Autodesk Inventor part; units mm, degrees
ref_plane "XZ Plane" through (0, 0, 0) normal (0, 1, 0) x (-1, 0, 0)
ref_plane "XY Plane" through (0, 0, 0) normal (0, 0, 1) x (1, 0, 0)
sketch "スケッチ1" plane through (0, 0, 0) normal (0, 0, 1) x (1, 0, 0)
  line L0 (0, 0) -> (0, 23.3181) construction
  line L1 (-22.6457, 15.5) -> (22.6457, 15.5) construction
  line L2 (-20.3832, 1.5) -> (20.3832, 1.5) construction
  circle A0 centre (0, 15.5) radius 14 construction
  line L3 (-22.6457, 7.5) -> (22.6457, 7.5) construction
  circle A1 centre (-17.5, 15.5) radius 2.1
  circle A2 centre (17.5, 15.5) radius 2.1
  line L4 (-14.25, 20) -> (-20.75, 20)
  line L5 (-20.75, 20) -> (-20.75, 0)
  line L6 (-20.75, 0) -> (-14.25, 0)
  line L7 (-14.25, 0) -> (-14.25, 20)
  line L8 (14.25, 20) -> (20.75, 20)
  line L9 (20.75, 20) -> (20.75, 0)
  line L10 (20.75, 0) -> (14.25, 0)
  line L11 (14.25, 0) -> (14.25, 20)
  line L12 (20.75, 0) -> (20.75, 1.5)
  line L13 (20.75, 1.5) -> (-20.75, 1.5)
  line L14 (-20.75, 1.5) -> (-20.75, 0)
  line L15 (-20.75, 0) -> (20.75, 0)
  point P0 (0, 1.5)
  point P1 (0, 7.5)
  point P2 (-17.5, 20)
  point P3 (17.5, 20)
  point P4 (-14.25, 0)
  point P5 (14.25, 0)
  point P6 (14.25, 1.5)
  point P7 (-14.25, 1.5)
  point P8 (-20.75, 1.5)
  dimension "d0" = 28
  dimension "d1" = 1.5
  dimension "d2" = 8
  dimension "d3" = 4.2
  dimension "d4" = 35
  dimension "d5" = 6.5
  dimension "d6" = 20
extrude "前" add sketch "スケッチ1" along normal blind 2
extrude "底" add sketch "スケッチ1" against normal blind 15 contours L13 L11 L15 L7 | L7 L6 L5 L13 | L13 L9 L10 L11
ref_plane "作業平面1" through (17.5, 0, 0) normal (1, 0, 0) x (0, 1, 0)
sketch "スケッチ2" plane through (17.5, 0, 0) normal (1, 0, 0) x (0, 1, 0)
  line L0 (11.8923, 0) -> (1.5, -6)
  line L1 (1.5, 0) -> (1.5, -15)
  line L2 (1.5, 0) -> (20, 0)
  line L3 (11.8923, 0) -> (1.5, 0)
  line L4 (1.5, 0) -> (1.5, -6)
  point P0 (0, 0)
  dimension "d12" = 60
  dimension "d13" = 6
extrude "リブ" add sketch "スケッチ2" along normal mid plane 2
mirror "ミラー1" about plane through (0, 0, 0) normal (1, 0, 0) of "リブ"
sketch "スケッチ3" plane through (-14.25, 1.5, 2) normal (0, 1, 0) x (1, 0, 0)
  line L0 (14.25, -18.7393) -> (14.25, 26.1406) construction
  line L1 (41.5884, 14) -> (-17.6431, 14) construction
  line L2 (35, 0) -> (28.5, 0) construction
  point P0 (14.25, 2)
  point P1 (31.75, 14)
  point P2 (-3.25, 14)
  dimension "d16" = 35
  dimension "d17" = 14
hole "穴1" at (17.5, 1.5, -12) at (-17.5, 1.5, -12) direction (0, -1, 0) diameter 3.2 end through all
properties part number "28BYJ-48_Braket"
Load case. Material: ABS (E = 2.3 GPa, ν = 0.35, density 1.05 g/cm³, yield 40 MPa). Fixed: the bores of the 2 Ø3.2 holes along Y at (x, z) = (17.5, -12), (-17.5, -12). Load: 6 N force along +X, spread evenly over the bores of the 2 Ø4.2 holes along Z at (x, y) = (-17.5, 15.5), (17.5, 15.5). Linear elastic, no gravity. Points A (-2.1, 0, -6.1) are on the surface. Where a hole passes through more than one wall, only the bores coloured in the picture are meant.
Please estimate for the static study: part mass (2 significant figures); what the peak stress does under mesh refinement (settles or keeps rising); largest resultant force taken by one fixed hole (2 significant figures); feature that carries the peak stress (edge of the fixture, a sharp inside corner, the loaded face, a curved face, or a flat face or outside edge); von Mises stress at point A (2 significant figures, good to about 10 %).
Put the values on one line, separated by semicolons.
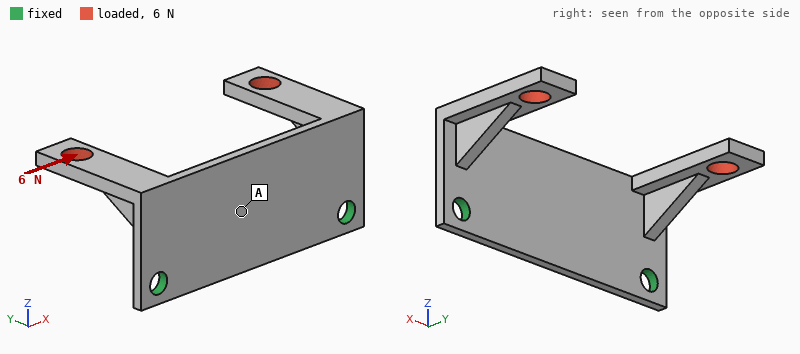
1.7 g; keeps rising; 3.8 N; edge of the fixture; 1.0 MPa
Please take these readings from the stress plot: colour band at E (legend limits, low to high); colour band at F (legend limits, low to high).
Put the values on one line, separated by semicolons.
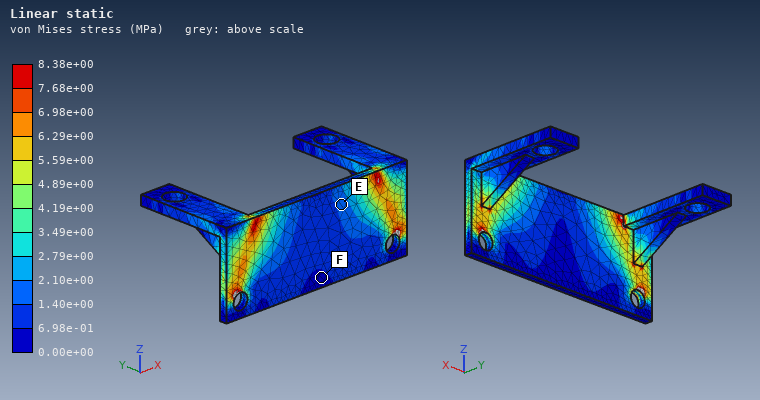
1.40e+00 to 2.10e+00 MPa; 0.00e+00 to 6.98e-01 MPa
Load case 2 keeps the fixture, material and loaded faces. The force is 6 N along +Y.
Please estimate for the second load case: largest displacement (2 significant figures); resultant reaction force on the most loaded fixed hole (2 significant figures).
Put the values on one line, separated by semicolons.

0.51 mm; 3.0 N
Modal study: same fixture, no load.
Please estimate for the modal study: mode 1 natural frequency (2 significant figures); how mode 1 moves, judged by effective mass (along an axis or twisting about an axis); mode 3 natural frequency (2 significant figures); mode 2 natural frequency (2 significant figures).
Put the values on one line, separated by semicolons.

690 Hz; along Y; 990 Hz; 820 Hz
